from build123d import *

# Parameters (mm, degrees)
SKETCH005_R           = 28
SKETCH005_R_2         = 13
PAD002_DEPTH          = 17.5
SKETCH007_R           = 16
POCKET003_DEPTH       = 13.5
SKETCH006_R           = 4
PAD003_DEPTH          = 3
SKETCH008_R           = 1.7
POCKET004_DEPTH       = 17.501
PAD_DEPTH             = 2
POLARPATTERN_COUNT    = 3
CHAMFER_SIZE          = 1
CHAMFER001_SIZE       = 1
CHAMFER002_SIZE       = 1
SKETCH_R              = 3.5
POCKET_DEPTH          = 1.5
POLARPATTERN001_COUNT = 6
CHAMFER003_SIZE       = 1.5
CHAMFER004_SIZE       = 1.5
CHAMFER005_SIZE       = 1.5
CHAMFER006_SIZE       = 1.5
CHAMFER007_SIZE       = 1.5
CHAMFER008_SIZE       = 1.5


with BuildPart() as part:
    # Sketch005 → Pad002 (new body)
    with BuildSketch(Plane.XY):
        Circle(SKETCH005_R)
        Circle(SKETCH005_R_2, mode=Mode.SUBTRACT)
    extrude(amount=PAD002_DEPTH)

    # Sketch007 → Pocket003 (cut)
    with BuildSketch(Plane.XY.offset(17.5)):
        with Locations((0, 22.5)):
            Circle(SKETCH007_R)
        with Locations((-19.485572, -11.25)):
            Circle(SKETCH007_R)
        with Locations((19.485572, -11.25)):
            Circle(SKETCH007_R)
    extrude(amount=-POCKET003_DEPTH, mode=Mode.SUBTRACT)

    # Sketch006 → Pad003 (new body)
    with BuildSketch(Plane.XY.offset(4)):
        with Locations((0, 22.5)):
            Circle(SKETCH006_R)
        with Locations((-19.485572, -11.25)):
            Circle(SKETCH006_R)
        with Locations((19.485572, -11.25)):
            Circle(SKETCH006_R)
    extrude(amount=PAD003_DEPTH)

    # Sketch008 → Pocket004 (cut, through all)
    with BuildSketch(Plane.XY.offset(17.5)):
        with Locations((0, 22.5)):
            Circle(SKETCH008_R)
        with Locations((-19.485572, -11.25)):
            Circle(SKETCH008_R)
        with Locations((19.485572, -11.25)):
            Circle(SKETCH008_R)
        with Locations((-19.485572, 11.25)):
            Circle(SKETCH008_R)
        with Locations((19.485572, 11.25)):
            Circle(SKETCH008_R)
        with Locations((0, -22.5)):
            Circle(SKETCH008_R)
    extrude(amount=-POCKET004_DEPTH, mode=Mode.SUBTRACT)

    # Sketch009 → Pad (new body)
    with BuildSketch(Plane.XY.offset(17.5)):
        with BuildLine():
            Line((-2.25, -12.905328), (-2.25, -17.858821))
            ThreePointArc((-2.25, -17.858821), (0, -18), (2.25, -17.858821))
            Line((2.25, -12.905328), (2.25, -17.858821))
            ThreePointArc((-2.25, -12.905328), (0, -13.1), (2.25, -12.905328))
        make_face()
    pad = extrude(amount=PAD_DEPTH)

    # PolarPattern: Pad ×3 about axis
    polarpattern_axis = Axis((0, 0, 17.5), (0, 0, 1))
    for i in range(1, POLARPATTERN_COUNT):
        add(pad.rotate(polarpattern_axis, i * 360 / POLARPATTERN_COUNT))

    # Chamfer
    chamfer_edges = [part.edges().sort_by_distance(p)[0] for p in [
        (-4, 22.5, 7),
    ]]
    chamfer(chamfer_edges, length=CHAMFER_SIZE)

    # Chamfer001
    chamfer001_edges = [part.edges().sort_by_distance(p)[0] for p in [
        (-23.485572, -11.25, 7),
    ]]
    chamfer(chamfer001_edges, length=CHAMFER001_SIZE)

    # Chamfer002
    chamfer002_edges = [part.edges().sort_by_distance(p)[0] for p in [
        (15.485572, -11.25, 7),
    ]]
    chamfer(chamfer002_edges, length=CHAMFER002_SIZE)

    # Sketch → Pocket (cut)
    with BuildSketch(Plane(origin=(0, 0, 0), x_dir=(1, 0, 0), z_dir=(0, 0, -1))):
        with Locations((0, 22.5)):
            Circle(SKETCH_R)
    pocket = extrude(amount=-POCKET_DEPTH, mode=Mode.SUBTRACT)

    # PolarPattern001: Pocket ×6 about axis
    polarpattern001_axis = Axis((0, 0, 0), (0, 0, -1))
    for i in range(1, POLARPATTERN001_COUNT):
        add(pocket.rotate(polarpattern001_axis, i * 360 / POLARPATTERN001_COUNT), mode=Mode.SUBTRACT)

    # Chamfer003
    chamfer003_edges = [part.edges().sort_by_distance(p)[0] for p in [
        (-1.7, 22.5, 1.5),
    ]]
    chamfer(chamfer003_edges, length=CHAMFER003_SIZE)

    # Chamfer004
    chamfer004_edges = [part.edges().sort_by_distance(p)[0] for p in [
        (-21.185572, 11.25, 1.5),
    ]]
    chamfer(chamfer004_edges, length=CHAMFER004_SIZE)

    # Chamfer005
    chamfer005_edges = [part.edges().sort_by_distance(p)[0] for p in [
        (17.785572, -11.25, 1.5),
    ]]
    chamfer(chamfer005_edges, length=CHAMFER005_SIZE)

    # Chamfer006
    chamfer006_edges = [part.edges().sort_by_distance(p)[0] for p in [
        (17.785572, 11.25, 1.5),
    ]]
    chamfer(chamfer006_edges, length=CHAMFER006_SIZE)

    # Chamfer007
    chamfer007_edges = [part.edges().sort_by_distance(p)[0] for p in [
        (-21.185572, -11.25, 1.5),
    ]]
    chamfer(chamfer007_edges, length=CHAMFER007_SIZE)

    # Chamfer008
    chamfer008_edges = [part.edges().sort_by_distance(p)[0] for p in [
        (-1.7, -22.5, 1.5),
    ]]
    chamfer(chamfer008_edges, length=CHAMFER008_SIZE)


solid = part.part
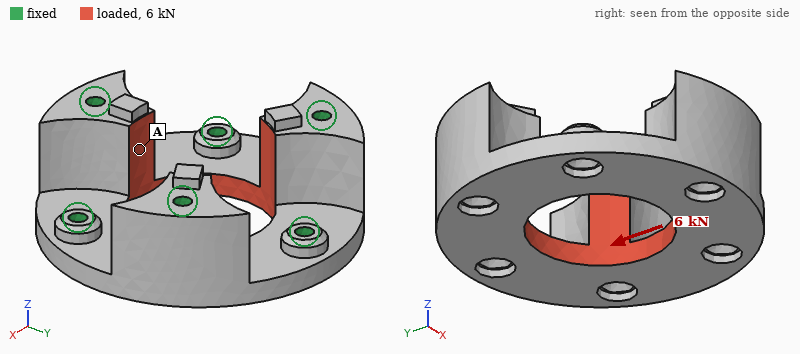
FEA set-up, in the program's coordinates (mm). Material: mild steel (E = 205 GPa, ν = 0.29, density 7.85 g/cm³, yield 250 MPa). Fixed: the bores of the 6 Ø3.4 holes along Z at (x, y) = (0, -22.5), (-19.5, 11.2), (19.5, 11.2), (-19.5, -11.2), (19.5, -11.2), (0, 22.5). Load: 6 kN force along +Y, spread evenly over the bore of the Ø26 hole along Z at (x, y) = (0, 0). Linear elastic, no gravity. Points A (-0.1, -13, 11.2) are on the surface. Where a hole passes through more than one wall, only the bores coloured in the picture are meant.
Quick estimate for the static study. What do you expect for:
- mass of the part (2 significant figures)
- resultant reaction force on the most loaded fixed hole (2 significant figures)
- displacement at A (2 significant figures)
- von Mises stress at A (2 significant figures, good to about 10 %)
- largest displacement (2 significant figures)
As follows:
120 g
1.6 kN
0.46 µm
9.6 MPa
2.6 µm
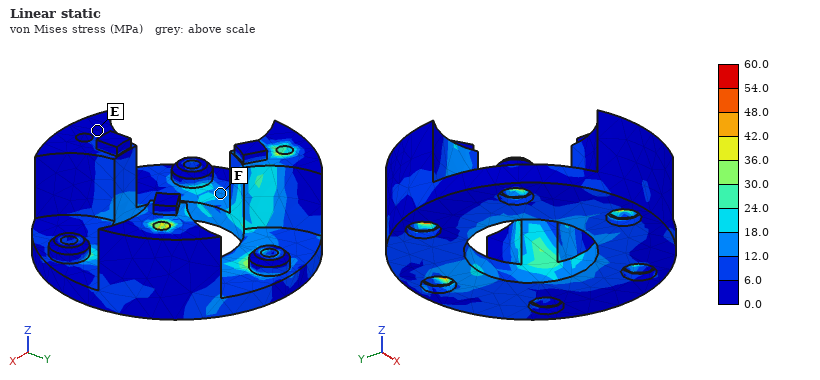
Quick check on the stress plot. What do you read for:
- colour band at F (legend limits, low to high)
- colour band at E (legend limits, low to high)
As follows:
12.0 to 18.0 MPa
0.0 to 6.0 MPa
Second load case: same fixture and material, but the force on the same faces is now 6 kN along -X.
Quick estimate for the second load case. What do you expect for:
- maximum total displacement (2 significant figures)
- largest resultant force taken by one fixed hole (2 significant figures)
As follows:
2.9 µm
1.6 kN
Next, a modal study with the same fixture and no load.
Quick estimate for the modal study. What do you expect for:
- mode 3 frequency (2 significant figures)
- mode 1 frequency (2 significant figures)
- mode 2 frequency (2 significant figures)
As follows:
41 kHz
40 kHz
40 kHz
